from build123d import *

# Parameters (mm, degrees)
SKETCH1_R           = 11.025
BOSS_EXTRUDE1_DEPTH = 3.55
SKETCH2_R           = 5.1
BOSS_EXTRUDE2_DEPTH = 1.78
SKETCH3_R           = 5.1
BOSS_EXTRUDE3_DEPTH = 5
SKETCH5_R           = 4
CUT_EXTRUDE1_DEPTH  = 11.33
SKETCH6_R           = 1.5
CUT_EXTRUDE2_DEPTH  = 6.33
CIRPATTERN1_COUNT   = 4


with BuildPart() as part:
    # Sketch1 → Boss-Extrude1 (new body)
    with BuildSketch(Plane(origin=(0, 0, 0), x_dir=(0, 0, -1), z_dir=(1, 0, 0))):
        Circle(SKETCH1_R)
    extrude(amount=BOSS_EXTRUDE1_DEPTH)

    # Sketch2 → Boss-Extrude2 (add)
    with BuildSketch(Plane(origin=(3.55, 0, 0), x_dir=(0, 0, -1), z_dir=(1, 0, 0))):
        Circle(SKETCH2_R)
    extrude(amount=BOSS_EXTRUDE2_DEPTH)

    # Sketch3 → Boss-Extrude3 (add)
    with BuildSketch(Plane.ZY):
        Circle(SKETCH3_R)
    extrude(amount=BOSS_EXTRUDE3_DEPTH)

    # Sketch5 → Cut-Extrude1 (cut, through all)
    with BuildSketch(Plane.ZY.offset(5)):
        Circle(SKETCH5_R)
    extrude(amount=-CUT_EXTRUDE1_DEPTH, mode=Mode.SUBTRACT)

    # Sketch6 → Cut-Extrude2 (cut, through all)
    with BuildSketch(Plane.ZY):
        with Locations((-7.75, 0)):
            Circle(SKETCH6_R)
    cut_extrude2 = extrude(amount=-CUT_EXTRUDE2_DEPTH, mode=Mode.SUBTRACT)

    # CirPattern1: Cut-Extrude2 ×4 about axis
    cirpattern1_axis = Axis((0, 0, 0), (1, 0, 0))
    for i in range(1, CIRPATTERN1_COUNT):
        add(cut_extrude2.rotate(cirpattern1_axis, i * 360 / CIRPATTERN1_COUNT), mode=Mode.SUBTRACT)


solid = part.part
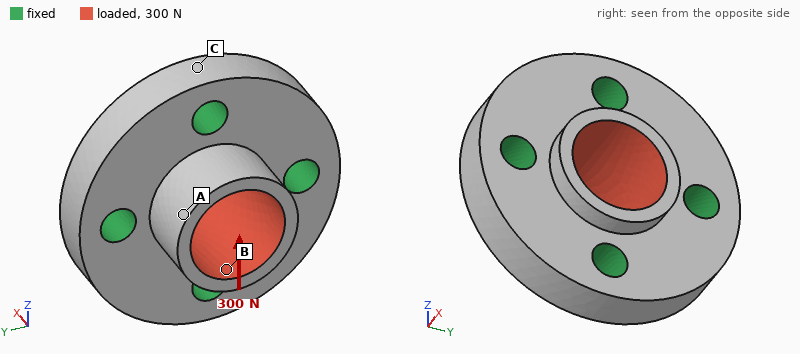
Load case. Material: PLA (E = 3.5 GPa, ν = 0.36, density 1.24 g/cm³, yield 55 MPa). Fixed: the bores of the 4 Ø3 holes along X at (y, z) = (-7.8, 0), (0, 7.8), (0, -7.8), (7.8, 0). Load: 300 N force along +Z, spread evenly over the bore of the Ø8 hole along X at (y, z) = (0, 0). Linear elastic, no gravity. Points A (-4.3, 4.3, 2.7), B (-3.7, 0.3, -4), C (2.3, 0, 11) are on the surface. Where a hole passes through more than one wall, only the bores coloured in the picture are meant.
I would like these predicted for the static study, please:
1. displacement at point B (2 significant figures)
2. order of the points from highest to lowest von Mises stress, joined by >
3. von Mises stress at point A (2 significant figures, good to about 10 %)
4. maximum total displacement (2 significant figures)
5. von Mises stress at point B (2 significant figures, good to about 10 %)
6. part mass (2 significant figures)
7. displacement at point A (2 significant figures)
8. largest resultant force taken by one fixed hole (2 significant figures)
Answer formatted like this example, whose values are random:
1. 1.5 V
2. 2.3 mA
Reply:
1. 30 µm
2. B > A > C
3. 3.4 MPa
4. 36 µm
5. 5.8 MPa
6. 1.6 g
7. 28 µm
8. 90 N
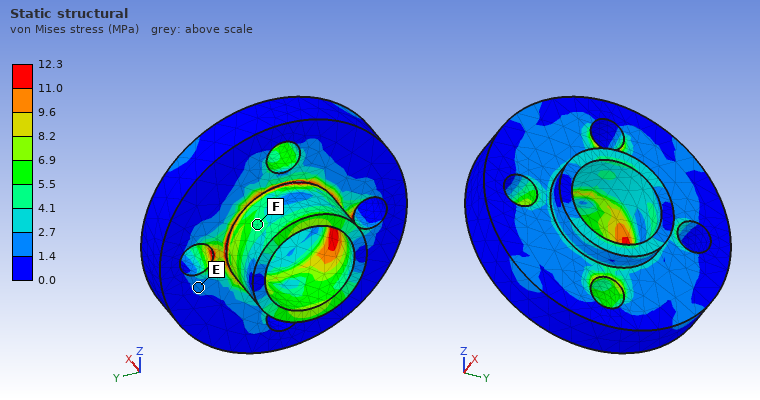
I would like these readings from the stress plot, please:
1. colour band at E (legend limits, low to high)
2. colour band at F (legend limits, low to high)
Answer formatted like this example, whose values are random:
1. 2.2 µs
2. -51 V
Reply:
1. 1.4 to 2.7 MPa
2. 4.1 to 5.5 MPa
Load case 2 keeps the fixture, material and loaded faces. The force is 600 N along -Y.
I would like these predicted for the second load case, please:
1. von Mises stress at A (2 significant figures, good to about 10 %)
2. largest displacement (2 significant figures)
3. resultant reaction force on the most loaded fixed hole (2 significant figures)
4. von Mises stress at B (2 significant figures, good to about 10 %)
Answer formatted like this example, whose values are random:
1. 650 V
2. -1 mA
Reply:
1. 9.3 MPa
2. 72 µm
3. 180 N
4. 13 MPa
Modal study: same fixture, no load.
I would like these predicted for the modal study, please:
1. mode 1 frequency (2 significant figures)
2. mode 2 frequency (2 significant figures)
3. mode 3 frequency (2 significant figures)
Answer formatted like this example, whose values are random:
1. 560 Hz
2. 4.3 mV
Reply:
1. 23 kHz
2. 24 kHz
3. 27 kHz
